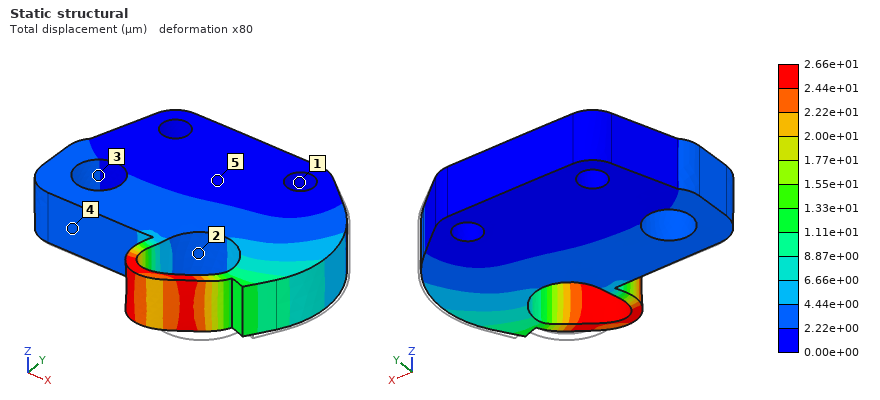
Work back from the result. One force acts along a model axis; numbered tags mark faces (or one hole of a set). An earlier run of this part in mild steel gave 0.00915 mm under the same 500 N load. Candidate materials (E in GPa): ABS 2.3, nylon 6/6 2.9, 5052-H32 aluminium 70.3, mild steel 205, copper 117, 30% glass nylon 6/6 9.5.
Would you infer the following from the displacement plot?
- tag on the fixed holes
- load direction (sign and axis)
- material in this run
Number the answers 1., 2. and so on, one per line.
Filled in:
1. 1
2. -X
3. 5052-H32 aluminium
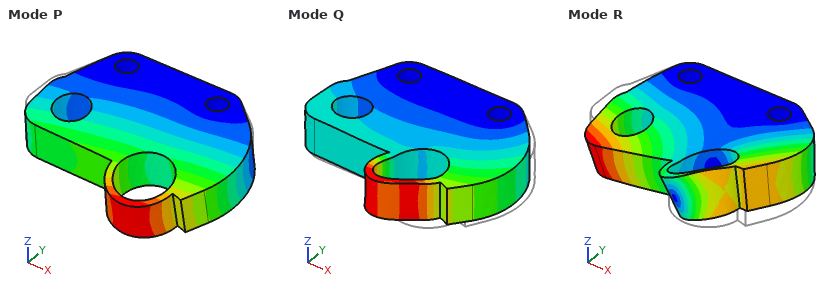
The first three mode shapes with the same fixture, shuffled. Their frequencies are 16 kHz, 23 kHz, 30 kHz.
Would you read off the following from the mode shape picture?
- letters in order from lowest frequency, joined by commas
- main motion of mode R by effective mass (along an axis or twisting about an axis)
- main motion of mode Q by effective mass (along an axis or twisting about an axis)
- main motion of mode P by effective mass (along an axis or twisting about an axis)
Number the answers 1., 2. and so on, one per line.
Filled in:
1. P, R, Q
2. twisting about Y
3. along X
4. along Z
